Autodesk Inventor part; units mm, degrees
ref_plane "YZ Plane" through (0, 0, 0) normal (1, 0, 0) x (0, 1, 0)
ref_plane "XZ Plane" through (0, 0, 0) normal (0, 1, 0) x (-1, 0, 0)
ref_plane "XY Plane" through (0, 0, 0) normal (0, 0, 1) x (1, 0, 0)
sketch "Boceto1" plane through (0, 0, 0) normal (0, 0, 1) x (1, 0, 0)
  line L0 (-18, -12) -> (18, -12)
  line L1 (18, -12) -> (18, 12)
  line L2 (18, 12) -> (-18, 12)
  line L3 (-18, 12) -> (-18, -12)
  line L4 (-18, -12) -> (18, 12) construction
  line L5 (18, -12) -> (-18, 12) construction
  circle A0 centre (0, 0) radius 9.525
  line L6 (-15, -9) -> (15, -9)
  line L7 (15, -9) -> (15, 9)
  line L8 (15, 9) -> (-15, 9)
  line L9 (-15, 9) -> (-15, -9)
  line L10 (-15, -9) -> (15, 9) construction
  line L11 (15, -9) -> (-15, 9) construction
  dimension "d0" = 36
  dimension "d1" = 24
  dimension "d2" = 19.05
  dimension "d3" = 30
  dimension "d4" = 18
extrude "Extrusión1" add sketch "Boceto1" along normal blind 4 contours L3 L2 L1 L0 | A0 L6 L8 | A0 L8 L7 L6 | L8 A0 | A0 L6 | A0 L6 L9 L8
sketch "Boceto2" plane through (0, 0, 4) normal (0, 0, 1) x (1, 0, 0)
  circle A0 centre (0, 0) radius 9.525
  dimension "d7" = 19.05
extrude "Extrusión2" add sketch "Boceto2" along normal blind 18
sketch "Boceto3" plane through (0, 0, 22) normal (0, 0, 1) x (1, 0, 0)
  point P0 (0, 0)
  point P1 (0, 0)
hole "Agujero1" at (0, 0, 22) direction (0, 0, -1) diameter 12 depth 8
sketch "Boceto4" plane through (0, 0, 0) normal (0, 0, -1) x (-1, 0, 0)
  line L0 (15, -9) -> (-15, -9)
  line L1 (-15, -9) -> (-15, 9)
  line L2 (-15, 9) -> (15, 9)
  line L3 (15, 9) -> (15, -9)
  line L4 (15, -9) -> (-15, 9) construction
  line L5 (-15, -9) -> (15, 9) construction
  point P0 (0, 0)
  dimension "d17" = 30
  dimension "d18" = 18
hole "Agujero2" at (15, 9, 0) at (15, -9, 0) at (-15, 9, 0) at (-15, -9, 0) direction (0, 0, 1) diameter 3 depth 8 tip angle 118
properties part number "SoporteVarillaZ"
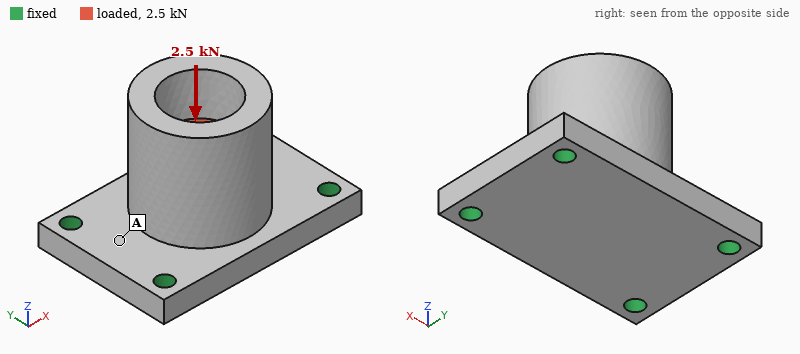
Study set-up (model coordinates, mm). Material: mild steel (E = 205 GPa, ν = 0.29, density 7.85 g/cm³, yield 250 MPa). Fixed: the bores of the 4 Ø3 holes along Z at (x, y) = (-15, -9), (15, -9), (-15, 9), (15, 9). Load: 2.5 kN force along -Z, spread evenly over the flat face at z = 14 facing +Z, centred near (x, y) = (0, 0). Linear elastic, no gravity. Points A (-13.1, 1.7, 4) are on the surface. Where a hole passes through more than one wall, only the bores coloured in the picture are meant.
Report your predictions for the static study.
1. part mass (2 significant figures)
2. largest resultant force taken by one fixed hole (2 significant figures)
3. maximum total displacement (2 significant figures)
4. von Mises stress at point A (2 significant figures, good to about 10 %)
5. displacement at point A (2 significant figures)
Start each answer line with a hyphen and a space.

- 59 g
- 660 N
- 7.0 µm
- 23 MPa
- 2.8 µm
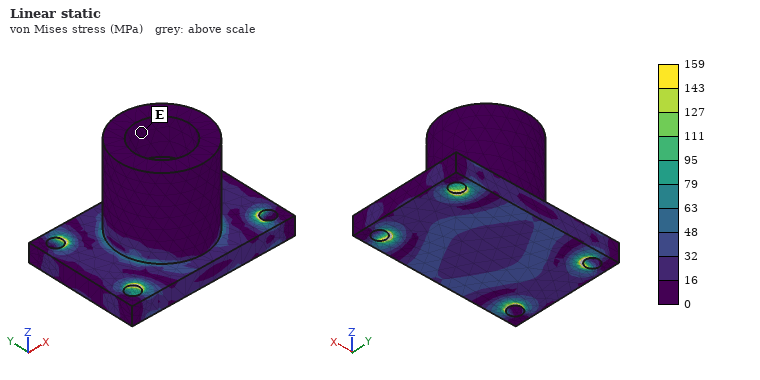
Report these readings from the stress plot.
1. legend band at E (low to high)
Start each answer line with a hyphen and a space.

- 0 to 16 MPa
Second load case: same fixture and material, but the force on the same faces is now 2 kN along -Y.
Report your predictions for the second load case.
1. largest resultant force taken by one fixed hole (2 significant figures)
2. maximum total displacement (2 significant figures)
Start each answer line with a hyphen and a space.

- 950 N
- 24 µm
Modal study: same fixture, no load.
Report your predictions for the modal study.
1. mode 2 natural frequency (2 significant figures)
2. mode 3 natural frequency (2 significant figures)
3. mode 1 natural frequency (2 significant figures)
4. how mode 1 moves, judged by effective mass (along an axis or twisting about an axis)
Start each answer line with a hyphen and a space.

- 15 kHz
- 15 kHz
- 10 kHz
- along Y
